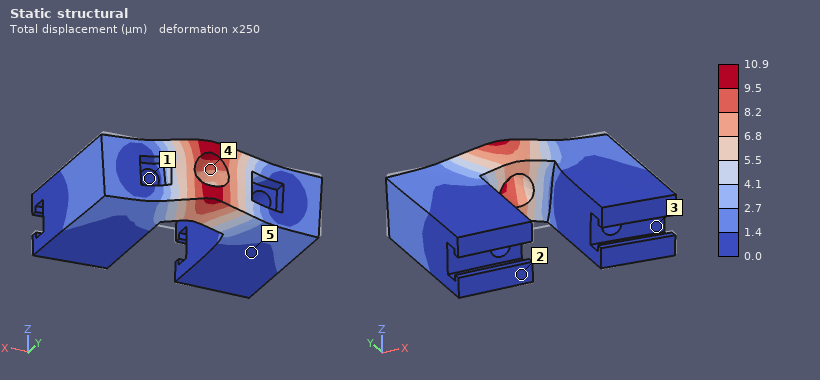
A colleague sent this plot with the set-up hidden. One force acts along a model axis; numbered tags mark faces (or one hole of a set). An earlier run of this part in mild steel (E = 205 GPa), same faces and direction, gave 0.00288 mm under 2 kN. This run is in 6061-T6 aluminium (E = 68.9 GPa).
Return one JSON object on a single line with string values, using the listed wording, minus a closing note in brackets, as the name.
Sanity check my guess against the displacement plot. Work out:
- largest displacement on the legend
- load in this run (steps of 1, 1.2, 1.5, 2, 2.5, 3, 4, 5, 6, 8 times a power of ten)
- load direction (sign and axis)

{"largest displacement on the legend": "10.9 µm", "load in this run": "2.5 kN", "load direction": "+Z"}
